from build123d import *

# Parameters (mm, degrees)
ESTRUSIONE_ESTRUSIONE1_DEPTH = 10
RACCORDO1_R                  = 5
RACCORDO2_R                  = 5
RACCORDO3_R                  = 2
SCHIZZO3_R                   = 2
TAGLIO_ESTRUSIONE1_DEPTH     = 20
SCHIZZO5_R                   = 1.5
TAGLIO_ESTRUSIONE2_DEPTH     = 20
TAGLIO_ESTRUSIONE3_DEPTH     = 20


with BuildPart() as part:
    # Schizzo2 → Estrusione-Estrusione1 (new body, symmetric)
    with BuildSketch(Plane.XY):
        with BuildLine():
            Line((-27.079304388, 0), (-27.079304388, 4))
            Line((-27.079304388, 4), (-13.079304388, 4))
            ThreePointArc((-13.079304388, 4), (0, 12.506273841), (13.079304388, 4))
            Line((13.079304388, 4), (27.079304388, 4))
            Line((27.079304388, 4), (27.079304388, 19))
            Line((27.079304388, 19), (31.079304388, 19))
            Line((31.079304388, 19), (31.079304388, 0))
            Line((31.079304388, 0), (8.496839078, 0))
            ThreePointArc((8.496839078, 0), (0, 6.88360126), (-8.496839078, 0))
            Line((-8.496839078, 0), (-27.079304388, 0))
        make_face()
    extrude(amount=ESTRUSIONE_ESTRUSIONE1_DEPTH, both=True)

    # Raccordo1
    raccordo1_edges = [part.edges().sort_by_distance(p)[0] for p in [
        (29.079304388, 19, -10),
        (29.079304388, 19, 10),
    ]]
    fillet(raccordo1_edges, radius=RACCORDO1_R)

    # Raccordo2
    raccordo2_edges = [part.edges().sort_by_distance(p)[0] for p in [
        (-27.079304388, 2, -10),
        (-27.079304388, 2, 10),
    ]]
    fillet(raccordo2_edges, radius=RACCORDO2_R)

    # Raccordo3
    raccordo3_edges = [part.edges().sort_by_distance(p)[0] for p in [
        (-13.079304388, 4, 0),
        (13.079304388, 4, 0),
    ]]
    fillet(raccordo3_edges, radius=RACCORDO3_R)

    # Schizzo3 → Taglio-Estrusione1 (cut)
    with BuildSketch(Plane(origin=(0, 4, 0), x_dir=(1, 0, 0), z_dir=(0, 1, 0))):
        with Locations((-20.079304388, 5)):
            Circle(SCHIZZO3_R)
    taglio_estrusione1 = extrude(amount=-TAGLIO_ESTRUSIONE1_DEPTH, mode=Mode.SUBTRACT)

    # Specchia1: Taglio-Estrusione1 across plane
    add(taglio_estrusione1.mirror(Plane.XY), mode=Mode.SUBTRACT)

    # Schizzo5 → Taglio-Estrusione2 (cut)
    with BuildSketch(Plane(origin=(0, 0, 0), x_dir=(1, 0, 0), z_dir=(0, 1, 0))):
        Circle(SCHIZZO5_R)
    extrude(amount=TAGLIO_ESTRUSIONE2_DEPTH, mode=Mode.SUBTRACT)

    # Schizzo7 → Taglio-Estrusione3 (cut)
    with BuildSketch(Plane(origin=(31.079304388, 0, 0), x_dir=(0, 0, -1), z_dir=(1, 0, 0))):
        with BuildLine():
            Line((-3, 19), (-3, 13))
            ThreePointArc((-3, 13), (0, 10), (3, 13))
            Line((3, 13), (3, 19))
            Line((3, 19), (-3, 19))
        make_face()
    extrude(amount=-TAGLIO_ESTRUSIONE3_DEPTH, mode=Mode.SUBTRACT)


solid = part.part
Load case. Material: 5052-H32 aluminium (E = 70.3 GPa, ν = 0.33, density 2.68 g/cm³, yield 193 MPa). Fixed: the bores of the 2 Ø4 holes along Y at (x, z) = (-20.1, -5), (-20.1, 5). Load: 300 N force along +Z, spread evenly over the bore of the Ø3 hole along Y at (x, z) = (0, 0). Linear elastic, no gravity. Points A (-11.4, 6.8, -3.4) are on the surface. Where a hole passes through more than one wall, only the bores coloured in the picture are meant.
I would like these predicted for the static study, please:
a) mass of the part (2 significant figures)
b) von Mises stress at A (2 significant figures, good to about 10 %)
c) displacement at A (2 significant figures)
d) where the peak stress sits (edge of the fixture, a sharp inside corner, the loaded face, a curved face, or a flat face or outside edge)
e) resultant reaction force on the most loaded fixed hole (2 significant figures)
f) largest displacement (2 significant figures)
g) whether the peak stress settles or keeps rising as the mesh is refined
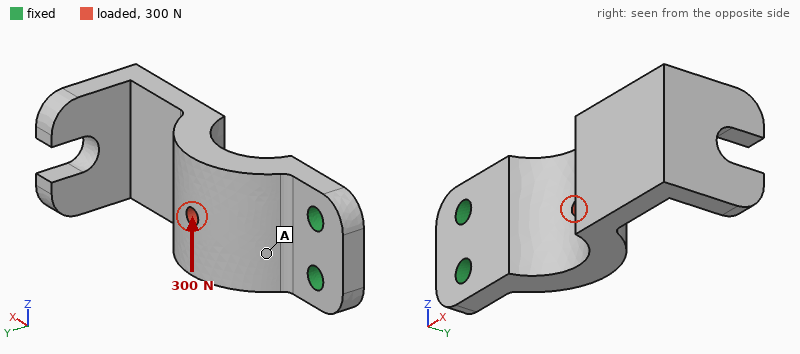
18 g
5.8 MPa
5.0 µm
edge of the fixture
510 N
26 µm
keeps rising
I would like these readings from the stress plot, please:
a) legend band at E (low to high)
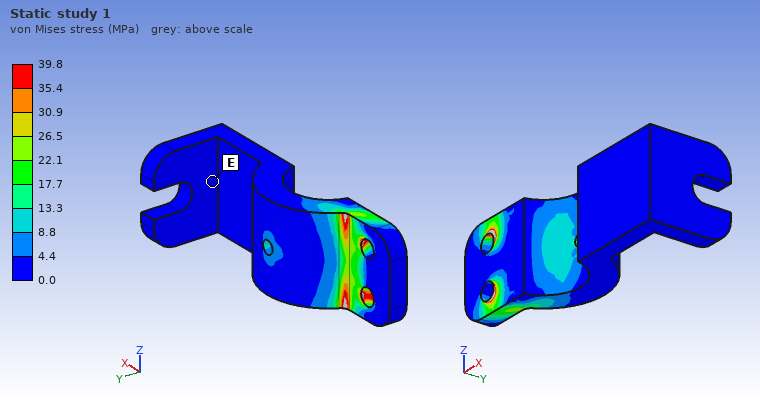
0.0 to 4.4 MPa
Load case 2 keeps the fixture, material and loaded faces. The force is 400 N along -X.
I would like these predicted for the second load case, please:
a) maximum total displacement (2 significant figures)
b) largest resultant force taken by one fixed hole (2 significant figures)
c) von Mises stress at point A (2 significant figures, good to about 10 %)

0.17 mm
210 N
16 MPa
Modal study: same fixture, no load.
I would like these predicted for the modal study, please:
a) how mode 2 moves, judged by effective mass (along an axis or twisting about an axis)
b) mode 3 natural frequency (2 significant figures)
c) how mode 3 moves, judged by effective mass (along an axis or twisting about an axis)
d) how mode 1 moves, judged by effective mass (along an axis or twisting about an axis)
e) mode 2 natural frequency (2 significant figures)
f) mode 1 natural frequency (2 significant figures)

along Z
5000 Hz
twisting about X
along Y
3000 Hz
1100 Hz
